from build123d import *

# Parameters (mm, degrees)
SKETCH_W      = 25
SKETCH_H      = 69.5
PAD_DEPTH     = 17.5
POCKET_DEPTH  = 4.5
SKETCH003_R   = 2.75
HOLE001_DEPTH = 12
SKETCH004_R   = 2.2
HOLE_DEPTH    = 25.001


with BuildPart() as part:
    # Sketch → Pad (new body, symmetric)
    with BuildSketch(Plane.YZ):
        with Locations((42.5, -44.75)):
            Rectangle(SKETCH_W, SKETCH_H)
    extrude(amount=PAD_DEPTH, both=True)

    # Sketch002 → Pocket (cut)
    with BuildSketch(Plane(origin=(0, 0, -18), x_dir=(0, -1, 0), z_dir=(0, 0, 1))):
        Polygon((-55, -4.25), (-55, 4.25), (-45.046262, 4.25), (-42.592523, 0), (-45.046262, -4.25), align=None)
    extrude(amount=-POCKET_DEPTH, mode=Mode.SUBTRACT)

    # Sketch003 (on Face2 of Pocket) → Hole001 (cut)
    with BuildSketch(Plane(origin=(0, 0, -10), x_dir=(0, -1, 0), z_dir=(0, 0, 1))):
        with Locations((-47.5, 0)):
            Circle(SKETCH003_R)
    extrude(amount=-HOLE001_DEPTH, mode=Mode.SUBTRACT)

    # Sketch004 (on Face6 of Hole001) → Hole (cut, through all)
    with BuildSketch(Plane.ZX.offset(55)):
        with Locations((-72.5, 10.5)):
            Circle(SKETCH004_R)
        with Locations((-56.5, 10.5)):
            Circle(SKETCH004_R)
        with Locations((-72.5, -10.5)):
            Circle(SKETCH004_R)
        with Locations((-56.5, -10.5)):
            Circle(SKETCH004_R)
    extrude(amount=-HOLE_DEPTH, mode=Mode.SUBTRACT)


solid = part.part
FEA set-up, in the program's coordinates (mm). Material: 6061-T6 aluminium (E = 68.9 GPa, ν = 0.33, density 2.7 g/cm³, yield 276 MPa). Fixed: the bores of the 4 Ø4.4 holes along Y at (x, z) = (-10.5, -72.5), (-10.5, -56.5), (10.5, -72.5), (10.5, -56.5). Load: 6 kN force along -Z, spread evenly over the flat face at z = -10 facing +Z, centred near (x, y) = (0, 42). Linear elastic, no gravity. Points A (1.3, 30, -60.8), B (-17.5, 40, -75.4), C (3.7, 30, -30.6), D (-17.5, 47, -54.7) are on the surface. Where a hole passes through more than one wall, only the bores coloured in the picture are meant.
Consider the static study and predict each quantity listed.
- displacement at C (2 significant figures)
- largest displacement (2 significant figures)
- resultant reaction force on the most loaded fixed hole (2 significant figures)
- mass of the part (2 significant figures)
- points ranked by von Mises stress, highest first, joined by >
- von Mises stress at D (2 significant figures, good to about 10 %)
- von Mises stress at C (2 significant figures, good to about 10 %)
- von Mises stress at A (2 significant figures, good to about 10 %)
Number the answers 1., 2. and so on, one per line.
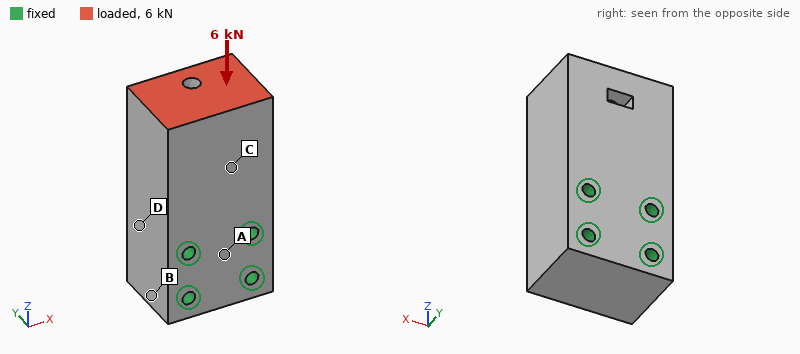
1. 2.8 µm
2. 5.9 µm
3. 2.6 kN
4. 160 g
5. C > D > A > B
6. 4.2 MPa
7. 7.0 MPa
8. 3.1 MPa
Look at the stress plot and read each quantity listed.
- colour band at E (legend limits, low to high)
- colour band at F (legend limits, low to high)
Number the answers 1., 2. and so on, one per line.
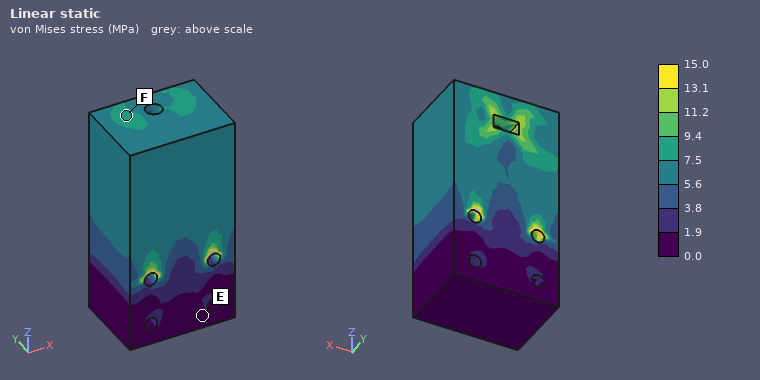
1. 0.0 to 1.9 MPa
2. 7.5 to 9.4 MPa
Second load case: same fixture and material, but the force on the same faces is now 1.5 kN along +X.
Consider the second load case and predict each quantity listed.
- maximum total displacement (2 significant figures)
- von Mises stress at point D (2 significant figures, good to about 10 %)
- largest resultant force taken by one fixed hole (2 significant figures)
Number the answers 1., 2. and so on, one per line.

1. 14 µm
2. 9.0 MPa
3. 2.7 kN
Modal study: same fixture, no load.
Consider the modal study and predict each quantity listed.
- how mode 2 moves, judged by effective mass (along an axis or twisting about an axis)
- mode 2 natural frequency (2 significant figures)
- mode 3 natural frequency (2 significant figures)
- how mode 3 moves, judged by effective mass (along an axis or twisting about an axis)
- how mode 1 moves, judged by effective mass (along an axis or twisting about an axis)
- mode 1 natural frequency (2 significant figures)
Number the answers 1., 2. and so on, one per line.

1. along X
2. 9600 Hz
3. 15 kHz
4. twisting about Z
5. along Y
6. 7700 Hz
